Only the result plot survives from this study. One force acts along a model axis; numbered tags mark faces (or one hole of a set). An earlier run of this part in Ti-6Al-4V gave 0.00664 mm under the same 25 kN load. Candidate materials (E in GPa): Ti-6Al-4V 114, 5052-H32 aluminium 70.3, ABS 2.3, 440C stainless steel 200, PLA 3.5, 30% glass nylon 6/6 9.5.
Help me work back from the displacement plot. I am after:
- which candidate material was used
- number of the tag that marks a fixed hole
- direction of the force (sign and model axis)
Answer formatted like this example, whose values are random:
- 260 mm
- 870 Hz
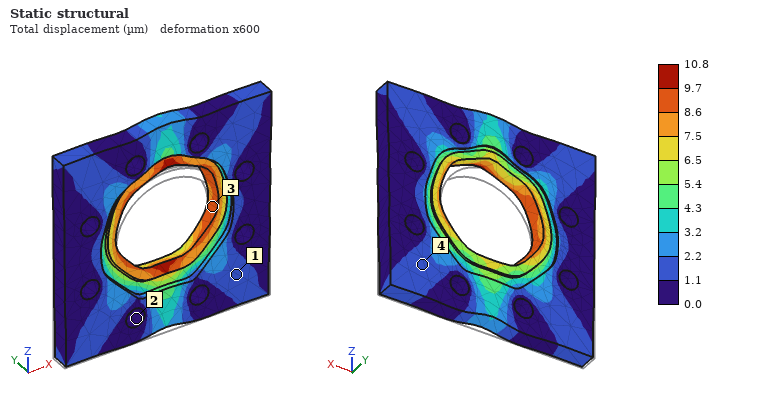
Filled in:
- 5052-H32 aluminium
- 2
- +Z
